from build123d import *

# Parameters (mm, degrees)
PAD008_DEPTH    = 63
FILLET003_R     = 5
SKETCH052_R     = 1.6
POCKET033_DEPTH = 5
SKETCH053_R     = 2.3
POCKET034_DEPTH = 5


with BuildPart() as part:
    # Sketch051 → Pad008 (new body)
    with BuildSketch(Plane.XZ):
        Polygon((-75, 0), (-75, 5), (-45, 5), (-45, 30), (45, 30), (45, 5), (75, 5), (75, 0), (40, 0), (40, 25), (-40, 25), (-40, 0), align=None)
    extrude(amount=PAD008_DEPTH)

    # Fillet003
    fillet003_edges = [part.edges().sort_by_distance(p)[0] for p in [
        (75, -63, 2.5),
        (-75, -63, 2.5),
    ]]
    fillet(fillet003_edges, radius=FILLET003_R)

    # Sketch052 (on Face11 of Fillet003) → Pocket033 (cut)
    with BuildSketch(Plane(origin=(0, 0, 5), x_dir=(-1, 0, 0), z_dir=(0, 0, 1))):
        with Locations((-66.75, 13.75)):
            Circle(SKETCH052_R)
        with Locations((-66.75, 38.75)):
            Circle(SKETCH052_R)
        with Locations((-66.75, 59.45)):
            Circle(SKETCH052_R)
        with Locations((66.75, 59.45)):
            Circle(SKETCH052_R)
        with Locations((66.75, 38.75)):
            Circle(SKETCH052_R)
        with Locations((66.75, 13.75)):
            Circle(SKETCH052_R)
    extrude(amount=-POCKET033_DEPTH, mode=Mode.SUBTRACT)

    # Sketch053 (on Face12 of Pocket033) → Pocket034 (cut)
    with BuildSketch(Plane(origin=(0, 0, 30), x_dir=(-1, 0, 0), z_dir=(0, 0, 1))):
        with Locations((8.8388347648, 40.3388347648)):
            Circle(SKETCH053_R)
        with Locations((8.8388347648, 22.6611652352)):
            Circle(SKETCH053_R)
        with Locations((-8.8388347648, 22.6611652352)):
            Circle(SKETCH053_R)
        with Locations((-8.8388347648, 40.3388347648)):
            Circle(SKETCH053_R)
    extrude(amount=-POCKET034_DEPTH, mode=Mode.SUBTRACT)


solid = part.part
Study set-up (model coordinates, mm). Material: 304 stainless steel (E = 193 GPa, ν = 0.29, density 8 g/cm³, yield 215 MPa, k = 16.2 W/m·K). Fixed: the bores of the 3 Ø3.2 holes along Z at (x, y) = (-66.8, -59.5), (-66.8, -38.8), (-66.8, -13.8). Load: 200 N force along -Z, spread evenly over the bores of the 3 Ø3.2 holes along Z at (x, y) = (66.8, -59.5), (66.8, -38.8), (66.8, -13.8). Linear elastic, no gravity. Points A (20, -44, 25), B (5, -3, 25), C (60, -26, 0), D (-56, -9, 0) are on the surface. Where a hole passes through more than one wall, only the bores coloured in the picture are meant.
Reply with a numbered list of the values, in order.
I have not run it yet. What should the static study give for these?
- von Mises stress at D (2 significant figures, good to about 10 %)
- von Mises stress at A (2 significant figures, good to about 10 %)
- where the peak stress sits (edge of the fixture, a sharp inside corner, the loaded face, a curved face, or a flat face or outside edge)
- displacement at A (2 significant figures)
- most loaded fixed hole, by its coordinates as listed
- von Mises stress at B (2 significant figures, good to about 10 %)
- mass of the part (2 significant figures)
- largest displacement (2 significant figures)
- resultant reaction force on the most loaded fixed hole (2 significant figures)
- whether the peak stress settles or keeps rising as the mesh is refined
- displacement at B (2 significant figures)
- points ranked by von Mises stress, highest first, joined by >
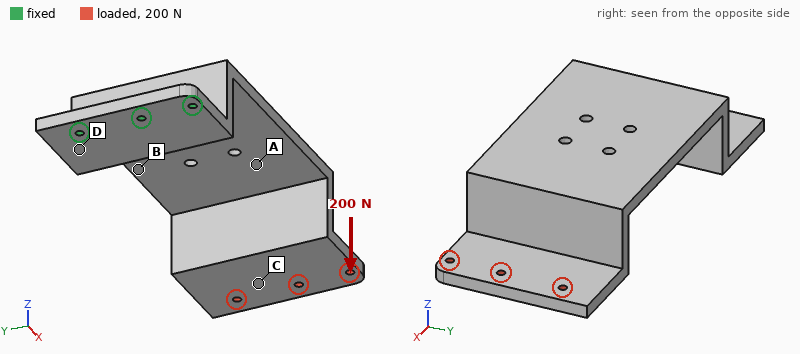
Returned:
1. 84 MPa
2. 33 MPa
3. edge of the fixture
4. 0.86 mm
5. (-66.8, -38.8)
6. 50 MPa
7. 500 g
8. 1.8 mm
9. 150 N
10. keeps rising
11. 0.62 mm
12. D > B > A > C
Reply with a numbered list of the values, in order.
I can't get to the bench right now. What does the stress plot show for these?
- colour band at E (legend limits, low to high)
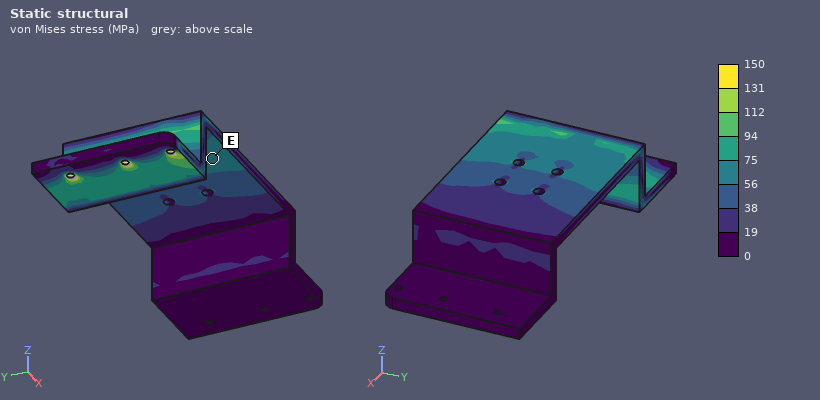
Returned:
1. 56 to 75 MPa
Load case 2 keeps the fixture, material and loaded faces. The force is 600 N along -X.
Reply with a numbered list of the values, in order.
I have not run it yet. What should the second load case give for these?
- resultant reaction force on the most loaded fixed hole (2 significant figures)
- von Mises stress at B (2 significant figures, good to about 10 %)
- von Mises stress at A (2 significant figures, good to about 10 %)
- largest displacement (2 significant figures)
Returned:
1. 200 N
2. 61 MPa
3. 55 MPa
4. 0.97 mm
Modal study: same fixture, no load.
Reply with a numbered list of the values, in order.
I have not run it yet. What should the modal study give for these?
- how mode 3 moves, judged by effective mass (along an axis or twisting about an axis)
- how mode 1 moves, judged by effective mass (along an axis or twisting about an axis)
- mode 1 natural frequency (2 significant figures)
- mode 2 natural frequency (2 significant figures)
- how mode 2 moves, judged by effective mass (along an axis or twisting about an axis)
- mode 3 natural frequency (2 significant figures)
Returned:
1. along X
2. along Z
3. 150 Hz
4. 390 Hz
5. along Y
6. 650 Hz
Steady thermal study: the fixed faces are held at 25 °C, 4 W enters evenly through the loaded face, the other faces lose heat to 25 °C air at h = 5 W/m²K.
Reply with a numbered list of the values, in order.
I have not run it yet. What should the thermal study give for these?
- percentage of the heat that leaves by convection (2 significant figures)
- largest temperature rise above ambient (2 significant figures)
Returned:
1. 79 %
2. 67 K
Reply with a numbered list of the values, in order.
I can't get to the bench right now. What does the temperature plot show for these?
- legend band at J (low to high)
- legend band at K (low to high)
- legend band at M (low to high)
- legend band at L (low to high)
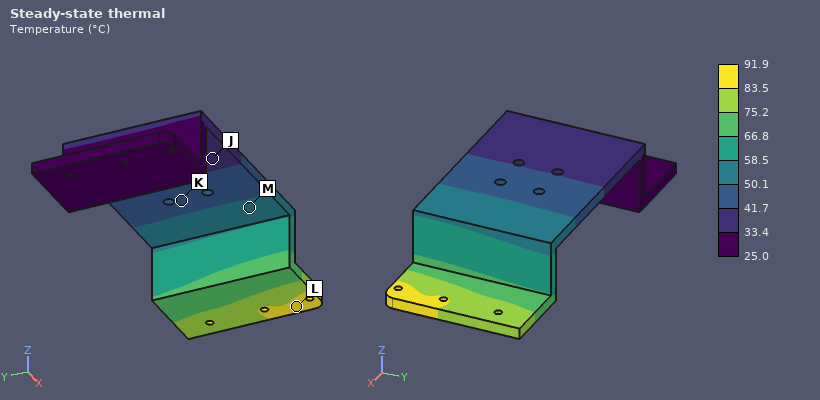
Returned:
1. 33.4 to 41.7 °C
2. 41.7 to 50.1 °C
3. 50.1 to 58.5 °C
4. 83.5 to 91.9 °C
